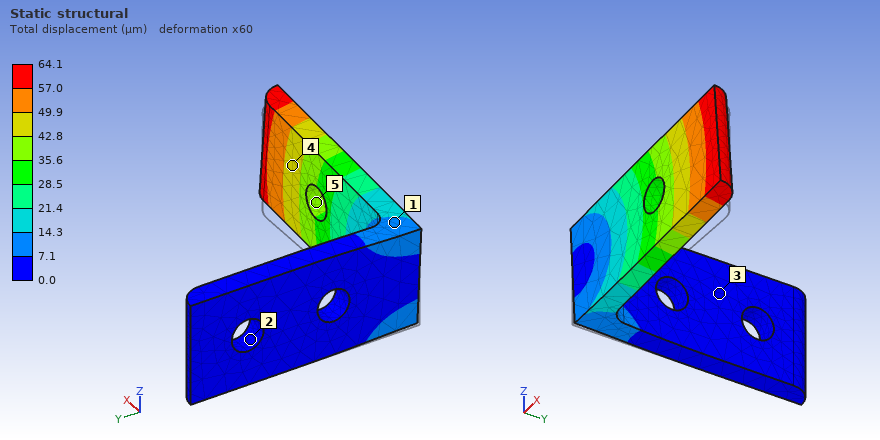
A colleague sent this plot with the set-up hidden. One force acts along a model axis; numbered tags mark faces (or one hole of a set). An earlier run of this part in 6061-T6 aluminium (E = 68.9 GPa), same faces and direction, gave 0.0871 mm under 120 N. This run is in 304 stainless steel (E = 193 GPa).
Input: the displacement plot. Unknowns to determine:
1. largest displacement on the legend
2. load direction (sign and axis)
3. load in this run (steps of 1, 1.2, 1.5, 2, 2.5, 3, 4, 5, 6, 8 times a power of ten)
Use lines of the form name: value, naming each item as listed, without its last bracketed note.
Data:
largest displacement on the legend: 64.1 µm
load direction: +Z
load in this run: 250 N
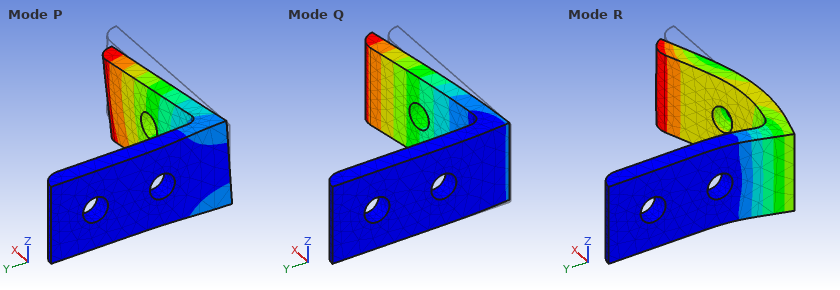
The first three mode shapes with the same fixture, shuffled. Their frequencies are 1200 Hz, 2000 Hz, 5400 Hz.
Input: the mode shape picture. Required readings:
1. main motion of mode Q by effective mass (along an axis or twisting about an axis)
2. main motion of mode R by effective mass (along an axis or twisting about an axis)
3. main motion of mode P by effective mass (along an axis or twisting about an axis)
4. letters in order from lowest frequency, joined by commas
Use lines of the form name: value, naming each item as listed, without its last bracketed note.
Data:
main motion of mode Q by effective mass: along Y
main motion of mode R by effective mass: along X
main motion of mode P by effective mass: along Z
letters in order from lowest frequency, joined by commas: Q, P, R
